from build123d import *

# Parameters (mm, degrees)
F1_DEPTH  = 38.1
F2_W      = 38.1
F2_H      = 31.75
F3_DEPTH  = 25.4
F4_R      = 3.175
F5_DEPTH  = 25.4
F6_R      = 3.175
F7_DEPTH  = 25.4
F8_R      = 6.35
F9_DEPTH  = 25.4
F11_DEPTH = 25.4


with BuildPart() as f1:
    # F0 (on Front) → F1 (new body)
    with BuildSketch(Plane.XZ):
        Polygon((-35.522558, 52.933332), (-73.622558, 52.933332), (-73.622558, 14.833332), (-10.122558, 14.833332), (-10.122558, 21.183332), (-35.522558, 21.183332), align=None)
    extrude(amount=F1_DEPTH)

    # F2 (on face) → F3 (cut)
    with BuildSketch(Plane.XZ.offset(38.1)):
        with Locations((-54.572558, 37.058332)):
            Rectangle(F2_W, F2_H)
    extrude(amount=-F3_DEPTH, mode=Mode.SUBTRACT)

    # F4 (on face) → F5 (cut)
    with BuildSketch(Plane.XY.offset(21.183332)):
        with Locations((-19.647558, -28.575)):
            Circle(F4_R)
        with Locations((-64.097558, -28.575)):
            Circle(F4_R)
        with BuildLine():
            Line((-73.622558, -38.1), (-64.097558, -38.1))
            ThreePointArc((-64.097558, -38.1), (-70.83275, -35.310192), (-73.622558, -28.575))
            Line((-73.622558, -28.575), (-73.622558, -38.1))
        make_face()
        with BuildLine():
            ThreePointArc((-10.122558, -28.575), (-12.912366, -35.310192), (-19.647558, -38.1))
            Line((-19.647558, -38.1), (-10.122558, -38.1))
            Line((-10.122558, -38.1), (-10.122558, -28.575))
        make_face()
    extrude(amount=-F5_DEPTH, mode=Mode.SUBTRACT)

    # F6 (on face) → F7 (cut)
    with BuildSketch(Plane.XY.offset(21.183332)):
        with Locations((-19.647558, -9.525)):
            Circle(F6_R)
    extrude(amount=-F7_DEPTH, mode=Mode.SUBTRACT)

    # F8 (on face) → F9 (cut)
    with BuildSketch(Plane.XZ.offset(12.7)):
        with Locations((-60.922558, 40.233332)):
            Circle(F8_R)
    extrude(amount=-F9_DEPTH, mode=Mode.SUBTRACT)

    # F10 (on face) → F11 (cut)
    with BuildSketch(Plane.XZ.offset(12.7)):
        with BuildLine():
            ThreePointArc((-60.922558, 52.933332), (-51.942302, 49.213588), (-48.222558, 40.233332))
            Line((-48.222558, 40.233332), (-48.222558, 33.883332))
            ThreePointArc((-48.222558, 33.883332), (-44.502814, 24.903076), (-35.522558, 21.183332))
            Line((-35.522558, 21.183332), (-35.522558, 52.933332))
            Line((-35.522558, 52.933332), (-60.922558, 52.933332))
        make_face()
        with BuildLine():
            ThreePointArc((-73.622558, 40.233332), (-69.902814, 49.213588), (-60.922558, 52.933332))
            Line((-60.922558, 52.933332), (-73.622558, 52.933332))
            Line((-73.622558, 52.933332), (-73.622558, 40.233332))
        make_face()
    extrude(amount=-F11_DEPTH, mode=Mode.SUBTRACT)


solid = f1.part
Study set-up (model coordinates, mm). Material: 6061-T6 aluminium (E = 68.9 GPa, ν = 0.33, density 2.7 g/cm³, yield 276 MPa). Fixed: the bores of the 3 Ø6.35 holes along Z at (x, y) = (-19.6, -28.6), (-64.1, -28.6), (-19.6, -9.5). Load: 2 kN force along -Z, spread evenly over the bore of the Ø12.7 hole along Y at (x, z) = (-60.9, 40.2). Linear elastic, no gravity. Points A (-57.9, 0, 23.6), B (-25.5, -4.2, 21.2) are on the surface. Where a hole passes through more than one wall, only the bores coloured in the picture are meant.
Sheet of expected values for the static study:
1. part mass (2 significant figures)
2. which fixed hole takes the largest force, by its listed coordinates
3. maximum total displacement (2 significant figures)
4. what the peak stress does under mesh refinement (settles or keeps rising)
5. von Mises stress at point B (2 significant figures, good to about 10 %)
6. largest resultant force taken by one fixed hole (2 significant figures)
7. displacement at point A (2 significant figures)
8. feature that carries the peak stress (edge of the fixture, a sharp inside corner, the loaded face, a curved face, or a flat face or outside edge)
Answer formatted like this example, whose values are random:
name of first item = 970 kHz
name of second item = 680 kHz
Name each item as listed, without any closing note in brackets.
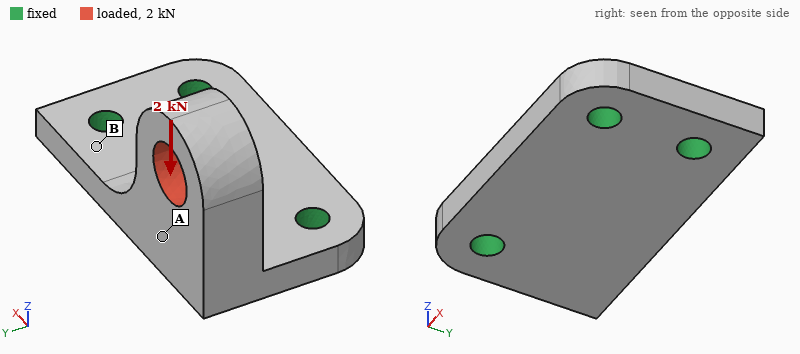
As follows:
part mass = 61 g
which fixed hole takes the largest force, by its listed coordinates = (-64.1, -28.6)
maximum total displacement = 0.22 mm
what the peak stress does under mesh refinement = keeps rising
von Mises stress at point B = 59 MPa
largest resultant force taken by one fixed hole = 1.6 kN
displacement at point A = 0.12 mm
feature that carries the peak stress = edge of the fixture
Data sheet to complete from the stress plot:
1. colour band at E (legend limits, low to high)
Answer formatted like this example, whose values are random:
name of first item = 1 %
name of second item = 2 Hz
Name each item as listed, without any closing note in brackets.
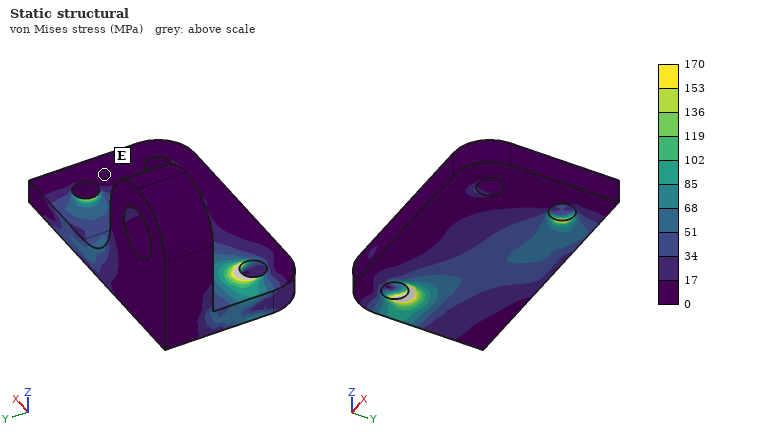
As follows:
colour band at E = 0 to 17 MPa
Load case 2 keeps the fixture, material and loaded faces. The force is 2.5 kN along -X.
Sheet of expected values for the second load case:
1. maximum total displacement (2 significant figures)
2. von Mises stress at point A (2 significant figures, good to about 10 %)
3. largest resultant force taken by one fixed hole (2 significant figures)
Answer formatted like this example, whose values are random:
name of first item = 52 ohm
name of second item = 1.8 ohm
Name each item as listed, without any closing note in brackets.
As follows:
maximum total displacement = 0.19 mm
von Mises stress at point A = 22 MPa
largest resultant force taken by one fixed hole = 1.6 kN
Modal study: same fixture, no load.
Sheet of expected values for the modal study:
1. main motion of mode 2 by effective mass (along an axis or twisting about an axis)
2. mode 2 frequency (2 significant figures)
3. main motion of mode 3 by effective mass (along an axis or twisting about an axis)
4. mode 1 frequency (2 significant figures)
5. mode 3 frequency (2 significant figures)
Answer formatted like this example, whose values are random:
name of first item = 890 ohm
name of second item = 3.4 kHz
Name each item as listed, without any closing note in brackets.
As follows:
main motion of mode 2 by effective mass = along X
mode 2 frequency = 6300 Hz
main motion of mode 3 by effective mass = along Z
mode 1 frequency = 2900 Hz
mode 3 frequency = 8800 Hz
